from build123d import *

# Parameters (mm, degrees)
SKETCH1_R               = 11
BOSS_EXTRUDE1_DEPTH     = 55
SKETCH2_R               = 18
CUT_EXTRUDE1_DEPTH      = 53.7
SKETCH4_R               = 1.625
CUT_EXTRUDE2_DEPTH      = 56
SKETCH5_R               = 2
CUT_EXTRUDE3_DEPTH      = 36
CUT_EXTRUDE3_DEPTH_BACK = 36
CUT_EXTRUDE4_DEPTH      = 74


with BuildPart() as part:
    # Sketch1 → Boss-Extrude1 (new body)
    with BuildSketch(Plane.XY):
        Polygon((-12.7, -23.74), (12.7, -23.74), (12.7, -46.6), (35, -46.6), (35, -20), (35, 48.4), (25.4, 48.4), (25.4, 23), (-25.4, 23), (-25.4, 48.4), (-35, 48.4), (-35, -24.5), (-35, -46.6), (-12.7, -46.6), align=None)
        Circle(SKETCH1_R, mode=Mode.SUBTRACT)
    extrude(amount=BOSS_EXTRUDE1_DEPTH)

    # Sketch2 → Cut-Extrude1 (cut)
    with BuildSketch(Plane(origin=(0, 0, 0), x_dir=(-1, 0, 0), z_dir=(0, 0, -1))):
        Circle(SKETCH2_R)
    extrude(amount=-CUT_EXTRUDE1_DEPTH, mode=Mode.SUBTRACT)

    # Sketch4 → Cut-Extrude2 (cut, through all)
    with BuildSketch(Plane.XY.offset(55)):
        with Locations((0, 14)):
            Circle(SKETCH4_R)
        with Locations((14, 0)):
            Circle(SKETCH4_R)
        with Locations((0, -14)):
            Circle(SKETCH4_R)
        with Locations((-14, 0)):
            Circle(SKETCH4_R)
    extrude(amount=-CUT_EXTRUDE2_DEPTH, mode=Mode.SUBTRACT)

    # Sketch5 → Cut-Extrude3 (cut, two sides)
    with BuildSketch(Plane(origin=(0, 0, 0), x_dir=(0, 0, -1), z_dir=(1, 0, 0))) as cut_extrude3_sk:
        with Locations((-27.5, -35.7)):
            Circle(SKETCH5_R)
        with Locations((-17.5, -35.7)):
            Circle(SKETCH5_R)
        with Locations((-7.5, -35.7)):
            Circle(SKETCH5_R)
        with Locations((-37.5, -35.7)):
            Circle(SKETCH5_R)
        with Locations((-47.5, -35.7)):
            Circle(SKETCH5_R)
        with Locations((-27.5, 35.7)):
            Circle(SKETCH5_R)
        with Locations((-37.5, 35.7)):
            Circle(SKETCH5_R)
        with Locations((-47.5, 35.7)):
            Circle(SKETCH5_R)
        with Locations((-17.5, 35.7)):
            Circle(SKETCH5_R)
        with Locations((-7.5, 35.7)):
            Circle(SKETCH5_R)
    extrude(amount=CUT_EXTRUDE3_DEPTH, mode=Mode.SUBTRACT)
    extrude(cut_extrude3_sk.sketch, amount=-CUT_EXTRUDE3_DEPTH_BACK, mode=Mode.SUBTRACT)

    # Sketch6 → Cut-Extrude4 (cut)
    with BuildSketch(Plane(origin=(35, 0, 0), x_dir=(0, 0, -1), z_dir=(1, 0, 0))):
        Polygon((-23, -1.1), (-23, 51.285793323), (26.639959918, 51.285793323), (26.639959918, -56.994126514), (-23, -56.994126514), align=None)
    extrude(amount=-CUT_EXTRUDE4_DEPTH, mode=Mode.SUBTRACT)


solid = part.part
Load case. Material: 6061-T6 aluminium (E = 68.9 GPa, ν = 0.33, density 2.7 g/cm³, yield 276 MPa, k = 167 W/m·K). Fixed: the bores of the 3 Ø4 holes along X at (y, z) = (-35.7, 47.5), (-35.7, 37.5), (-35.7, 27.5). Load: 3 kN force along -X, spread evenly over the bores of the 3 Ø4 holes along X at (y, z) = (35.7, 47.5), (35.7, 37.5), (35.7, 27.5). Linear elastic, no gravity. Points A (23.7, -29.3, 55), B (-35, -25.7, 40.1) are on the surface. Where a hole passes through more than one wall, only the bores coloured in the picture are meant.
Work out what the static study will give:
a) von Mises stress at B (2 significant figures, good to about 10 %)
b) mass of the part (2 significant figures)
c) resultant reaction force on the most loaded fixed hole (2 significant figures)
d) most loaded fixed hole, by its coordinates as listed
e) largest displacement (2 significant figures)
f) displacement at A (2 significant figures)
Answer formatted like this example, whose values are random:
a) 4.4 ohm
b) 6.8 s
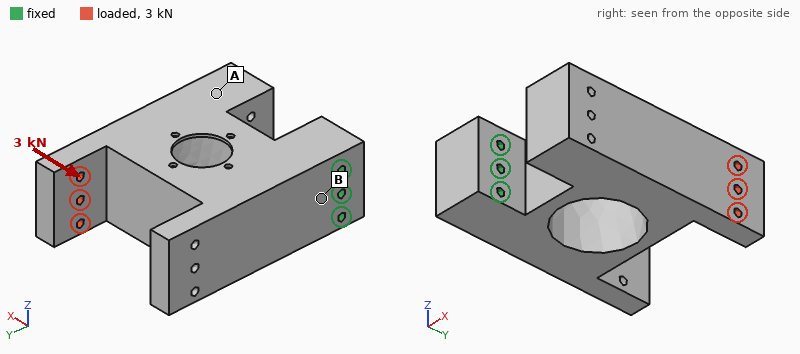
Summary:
a) 64 MPa
b) 320 g
c) 1.3 kN
d) (-35.7, 37.5)
e) 0.36 mm
f) 0.13 mm
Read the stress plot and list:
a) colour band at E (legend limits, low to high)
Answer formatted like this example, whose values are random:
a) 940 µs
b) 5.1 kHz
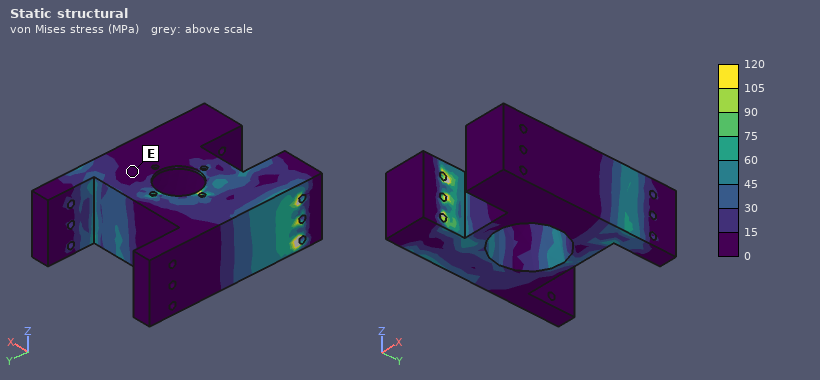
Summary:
a) 0 to 15 MPa
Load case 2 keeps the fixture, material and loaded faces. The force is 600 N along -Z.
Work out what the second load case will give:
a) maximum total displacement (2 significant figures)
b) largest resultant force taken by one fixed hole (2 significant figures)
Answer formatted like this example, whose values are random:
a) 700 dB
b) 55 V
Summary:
a) 96 µm
b) 2.2 kN
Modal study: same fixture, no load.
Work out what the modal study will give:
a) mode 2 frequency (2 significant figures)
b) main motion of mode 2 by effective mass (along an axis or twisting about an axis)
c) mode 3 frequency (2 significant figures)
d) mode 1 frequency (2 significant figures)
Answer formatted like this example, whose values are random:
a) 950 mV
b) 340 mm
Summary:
a) 1800 Hz
b) along Z
c) 2900 Hz
d) 1500 Hz
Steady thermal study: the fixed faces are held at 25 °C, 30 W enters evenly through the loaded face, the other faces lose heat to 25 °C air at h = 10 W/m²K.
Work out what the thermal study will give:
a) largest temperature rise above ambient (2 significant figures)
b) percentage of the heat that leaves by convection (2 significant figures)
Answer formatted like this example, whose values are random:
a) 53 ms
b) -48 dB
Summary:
a) 33 K
b) 11 %
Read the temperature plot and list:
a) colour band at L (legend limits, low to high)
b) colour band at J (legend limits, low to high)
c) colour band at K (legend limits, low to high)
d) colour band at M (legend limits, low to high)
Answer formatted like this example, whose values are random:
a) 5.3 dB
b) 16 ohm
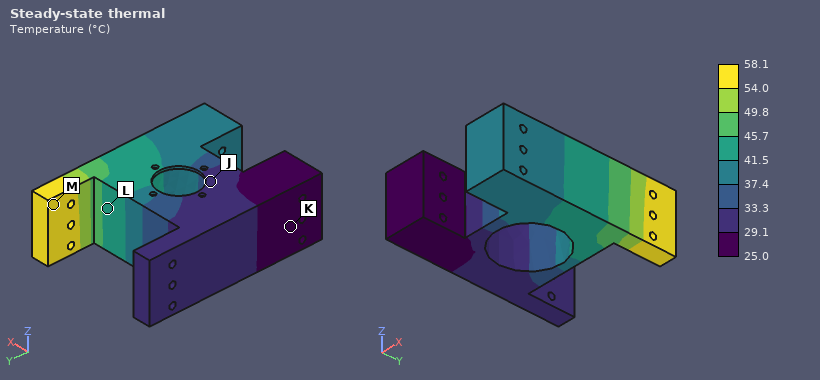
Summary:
a) 41.5 to 45.7 °C
b) 29.1 to 33.3 °C
c) 25.0 to 29.1 °C
d) 54.0 to 58.1 °C
